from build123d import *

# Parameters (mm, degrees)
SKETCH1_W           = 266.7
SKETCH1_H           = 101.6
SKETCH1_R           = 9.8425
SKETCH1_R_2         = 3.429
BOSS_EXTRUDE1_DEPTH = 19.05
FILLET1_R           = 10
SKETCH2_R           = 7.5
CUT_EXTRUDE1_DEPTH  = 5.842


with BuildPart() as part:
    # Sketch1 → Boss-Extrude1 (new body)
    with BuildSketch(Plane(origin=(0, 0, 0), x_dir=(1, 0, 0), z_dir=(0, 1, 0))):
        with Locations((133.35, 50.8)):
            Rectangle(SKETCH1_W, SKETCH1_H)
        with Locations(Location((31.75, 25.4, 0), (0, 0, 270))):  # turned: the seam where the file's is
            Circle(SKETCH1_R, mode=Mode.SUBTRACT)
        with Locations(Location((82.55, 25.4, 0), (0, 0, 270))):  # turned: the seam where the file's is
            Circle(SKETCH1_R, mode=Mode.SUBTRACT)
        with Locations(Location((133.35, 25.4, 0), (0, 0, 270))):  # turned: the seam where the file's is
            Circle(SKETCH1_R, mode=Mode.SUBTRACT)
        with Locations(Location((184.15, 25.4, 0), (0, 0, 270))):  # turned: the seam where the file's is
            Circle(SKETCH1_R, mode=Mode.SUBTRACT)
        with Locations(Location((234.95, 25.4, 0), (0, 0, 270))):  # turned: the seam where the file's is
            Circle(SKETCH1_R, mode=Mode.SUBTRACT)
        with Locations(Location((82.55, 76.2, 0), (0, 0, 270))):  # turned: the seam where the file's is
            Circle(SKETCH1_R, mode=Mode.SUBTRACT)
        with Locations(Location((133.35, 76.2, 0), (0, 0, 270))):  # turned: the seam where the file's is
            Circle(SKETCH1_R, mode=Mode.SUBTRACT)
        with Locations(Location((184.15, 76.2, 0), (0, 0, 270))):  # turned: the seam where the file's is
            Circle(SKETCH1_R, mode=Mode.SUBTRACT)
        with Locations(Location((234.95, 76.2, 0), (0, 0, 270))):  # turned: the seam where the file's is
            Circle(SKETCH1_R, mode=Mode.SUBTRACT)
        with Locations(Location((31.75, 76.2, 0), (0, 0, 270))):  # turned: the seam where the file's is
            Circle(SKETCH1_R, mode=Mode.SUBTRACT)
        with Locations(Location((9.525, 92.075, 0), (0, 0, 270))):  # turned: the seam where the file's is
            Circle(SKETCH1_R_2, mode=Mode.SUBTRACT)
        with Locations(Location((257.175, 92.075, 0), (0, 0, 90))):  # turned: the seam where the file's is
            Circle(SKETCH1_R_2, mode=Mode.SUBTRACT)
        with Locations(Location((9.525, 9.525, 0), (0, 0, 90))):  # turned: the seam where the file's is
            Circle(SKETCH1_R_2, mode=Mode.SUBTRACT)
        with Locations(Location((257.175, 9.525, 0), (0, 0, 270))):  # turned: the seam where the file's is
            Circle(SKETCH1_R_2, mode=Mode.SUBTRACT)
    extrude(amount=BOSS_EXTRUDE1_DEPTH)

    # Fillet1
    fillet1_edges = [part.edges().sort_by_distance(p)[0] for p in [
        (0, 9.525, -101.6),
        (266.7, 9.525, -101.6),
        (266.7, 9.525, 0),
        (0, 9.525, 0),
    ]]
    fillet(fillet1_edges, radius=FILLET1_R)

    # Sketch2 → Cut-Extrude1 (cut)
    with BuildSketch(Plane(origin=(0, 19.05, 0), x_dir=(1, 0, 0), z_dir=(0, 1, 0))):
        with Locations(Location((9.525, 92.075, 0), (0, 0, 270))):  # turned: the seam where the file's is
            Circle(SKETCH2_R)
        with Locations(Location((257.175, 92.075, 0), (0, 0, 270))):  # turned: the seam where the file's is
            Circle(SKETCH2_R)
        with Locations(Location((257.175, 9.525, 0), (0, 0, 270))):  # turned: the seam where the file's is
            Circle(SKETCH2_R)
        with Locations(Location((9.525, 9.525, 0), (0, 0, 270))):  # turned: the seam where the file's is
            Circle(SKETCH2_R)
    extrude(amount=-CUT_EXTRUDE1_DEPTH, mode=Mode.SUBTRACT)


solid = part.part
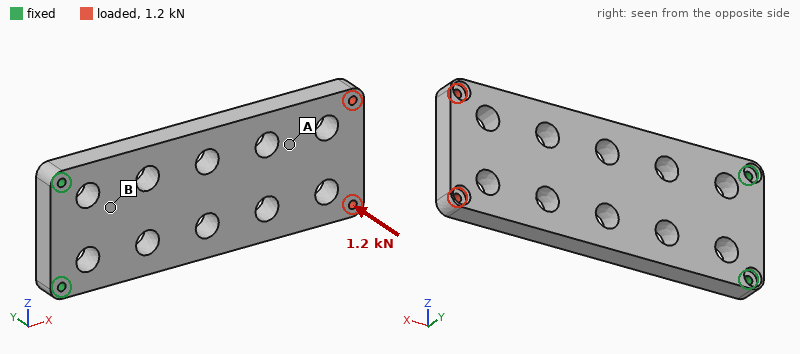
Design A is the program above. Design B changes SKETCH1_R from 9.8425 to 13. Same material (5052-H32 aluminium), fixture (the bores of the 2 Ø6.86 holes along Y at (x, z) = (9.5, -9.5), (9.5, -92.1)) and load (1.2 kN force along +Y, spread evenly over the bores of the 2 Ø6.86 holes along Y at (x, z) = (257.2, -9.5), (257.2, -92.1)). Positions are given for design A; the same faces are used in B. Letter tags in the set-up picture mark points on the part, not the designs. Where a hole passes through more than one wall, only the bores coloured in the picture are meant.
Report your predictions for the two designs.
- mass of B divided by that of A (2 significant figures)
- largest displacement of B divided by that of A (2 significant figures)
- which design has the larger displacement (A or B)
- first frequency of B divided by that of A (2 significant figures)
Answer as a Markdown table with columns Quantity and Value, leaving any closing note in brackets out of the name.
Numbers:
| Quantity | Value |
|---|---|
| mass of B divided by that of A | 0.90 |
| largest displacement of B divided by that of A | 1.2 |
| which design has the larger displacement | B |
| first frequency of B divided by that of A | 0.97 |
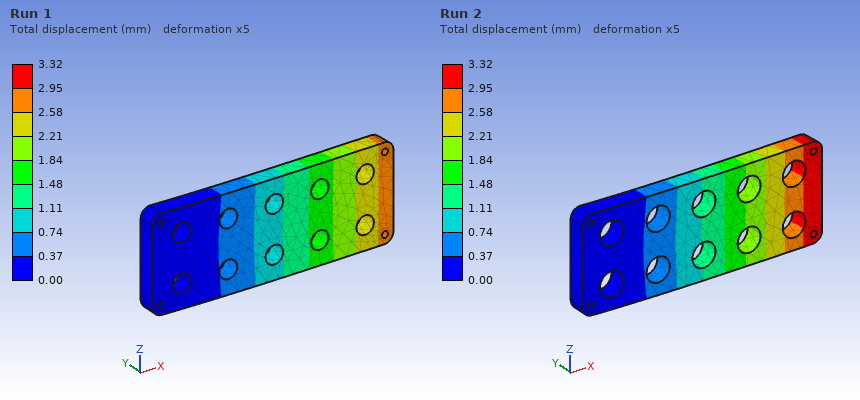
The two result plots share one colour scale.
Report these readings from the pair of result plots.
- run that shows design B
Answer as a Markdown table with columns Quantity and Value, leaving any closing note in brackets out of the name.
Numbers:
| Quantity | Value |
|---|---|
| run that shows design B | Run 2 |
